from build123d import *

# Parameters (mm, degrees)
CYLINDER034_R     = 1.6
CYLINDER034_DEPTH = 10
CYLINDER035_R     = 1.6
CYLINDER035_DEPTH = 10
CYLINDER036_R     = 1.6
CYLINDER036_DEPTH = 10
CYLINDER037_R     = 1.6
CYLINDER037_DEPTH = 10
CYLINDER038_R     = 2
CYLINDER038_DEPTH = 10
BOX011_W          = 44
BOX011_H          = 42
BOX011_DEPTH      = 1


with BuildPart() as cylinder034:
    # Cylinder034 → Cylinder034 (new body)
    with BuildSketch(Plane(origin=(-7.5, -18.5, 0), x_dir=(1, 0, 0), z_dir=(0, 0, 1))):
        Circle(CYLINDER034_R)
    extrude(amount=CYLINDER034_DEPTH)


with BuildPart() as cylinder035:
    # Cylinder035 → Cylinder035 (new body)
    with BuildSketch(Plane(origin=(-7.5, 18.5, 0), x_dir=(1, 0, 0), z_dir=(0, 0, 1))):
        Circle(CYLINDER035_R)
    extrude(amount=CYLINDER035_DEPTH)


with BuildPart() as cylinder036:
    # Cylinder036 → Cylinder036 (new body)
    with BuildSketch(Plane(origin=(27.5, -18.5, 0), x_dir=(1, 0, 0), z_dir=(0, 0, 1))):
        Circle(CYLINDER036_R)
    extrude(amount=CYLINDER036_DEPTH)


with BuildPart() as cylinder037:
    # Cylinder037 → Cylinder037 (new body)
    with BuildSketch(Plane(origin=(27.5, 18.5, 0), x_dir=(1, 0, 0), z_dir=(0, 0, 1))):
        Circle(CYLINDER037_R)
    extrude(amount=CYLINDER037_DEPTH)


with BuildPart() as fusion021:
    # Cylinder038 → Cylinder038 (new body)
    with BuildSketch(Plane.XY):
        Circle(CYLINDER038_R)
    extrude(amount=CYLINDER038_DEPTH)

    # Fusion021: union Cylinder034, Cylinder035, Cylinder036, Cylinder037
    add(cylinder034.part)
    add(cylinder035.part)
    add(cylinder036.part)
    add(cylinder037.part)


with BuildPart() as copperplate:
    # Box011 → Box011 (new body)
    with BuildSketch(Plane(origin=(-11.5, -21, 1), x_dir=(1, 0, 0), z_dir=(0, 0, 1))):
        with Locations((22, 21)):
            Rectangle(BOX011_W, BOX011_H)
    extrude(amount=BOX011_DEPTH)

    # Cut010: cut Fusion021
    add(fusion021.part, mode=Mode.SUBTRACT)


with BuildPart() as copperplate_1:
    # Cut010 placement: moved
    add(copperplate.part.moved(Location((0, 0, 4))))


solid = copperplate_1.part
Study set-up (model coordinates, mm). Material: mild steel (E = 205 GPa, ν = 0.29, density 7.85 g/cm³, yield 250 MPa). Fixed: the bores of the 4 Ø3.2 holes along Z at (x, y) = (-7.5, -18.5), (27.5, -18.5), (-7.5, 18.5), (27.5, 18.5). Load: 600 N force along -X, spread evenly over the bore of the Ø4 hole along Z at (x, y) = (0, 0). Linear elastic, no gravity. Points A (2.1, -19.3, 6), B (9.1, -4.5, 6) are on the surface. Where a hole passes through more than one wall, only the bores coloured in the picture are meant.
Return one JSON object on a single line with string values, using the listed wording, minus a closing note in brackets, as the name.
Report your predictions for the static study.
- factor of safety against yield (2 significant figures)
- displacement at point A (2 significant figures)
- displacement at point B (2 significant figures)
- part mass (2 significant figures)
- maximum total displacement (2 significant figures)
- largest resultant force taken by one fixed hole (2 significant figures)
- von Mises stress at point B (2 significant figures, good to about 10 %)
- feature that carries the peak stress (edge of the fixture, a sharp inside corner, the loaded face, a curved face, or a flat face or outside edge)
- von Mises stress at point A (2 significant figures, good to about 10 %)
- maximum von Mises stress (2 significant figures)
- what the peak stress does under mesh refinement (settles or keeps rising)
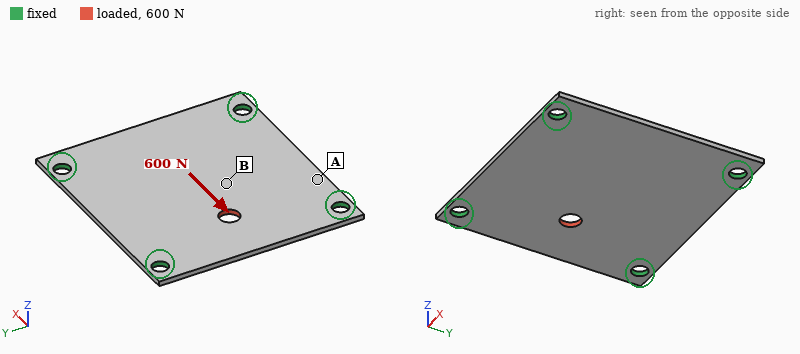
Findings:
{"factor of safety against yield": "2.8", "displacement at point A": "0.62 µm", "displacement at point B": "1.8 µm", "part mass": "14 g", "maximum total displacement": "3.8 µm", "largest resultant force taken by one fixed hole": "180 N", "von Mises stress at point B": "21 MPa", "feature that carries the peak stress": "the loaded face", "von Mises stress at point A": "9.6 MPa", "maximum von Mises stress": "89 MPa", "what the peak stress does under mesh refinement": "settles"}
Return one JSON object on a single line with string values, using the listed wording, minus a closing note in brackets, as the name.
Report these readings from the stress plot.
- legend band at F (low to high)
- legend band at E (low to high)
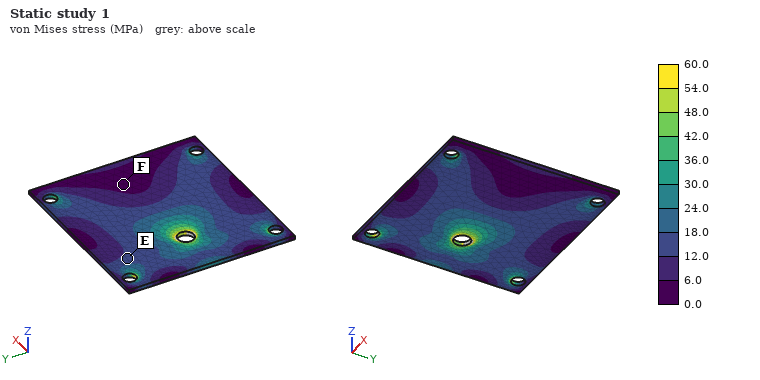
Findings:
{"legend band at F": "0.0 to 6.0 MPa", "legend band at E": "12.0 to 18.0 MPa"}
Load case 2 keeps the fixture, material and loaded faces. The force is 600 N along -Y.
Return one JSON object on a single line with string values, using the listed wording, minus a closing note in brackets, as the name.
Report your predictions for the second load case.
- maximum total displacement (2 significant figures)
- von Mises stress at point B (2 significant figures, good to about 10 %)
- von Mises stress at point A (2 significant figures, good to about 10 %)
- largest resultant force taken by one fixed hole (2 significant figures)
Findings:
{"maximum total displacement": "2.7 µm", "von Mises stress at point B": "8.6 MPa", "von Mises stress at point A": "7.1 MPa", "largest resultant force taken by one fixed hole": "230 N"}
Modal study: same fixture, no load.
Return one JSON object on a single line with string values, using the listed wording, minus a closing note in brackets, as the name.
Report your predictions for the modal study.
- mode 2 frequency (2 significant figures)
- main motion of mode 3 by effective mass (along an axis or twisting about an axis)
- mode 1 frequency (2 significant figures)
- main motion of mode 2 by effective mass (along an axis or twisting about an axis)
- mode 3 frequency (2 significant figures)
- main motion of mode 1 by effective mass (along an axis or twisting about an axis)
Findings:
{"mode 2 frequency": "4700 Hz", "main motion of mode 3 by effective mass": "twisting about X", "mode 1 frequency": "2900 Hz", "main motion of mode 2 by effective mass": "twisting about Y", "mode 3 frequency": "5200 Hz", "main motion of mode 1 by effective mass": "along Z"}
